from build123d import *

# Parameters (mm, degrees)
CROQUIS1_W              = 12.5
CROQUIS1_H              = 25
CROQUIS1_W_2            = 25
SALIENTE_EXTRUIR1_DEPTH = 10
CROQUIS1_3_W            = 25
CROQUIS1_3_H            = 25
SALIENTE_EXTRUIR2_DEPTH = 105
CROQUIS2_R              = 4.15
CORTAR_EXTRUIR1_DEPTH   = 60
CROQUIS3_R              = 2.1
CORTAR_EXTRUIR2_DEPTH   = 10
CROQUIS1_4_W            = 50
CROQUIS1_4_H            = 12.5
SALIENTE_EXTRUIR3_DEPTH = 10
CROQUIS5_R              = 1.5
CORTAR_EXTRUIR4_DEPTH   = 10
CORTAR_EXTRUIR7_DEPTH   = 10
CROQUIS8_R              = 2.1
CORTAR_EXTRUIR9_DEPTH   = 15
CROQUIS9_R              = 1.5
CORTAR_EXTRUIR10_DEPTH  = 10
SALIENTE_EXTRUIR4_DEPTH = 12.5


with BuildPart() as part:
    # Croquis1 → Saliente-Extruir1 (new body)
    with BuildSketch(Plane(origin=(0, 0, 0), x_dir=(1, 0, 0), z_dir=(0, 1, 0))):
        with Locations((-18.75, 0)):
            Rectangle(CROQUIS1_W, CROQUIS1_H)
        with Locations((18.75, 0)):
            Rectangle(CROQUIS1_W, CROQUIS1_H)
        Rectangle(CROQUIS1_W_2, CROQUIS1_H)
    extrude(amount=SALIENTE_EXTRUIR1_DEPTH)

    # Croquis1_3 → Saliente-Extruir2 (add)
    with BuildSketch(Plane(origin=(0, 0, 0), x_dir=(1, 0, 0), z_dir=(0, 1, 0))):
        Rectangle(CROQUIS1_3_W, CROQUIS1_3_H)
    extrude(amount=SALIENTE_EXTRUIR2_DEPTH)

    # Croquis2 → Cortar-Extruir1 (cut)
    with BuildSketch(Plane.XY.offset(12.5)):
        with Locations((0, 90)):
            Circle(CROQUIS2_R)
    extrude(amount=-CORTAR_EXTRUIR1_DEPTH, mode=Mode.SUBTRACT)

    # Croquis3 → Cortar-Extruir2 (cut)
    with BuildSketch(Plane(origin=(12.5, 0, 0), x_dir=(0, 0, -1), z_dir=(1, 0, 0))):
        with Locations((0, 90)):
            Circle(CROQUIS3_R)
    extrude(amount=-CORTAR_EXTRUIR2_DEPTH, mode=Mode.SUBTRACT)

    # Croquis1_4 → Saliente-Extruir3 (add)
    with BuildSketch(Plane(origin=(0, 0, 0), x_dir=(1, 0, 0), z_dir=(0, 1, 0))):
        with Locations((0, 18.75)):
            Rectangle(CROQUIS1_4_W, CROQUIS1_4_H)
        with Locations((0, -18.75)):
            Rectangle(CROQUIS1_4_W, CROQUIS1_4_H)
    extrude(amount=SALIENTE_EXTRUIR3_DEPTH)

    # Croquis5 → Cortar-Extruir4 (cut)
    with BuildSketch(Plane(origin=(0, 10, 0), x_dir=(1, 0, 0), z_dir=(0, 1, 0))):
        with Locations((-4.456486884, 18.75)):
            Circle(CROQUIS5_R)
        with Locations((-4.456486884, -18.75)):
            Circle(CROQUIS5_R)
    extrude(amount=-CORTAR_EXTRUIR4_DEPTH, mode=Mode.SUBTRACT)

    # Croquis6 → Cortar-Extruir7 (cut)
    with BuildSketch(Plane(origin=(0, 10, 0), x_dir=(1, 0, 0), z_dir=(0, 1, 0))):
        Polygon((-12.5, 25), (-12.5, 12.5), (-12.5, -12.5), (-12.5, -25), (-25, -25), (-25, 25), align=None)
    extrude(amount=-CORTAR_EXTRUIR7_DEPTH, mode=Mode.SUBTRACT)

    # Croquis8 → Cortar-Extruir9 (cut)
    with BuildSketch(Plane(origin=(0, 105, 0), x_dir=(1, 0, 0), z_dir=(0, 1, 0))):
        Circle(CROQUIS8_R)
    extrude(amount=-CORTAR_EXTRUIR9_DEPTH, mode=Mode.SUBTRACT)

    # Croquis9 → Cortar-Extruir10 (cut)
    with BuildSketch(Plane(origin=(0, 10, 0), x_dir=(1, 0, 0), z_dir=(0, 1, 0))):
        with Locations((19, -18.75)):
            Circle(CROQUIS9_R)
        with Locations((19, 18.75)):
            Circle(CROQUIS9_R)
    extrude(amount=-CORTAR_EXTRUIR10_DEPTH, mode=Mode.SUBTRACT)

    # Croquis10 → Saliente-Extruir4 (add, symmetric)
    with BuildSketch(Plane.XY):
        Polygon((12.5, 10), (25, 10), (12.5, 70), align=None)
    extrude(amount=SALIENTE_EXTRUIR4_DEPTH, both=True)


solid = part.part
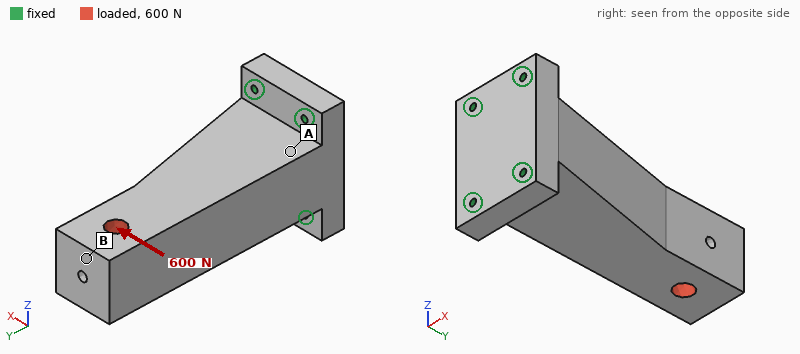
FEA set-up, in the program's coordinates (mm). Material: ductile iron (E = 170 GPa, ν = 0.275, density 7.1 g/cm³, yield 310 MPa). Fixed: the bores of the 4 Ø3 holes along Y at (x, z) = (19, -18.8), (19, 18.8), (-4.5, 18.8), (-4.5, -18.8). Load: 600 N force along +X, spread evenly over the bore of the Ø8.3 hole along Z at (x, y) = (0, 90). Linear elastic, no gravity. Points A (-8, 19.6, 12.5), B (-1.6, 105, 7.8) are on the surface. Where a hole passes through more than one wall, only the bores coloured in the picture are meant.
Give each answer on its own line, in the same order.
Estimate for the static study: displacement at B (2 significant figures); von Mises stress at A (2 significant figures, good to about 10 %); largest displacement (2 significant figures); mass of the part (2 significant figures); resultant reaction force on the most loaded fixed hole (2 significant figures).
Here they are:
26 µm
6.5 MPa
26 µm
610 g
970 N
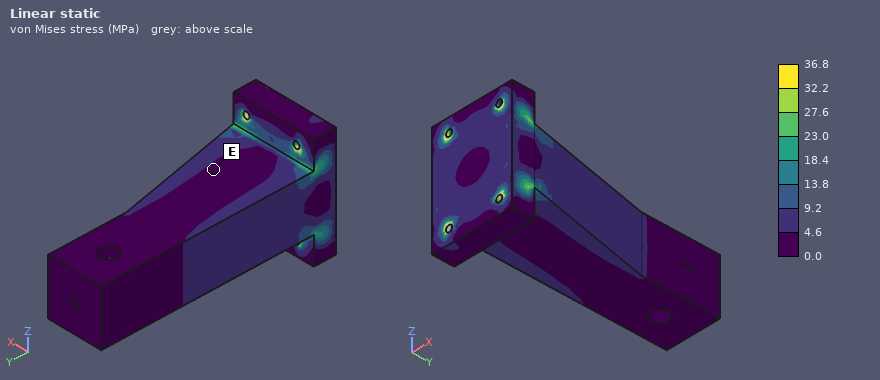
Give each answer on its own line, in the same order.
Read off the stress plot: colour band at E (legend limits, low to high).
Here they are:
0.0 to 4.6 MPa
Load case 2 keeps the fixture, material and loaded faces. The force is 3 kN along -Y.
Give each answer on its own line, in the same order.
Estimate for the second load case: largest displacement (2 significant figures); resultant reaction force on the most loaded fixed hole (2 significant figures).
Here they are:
9.7 µm
1.2 kN
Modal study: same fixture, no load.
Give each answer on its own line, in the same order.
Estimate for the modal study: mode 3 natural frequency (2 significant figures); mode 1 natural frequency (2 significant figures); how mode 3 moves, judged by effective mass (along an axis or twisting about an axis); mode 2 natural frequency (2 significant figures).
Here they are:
8400 Hz
2000 Hz
twisting about Y
2000 Hz
